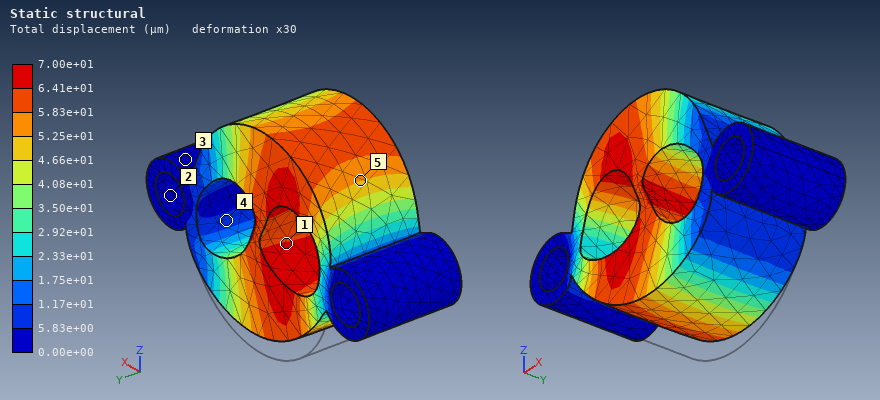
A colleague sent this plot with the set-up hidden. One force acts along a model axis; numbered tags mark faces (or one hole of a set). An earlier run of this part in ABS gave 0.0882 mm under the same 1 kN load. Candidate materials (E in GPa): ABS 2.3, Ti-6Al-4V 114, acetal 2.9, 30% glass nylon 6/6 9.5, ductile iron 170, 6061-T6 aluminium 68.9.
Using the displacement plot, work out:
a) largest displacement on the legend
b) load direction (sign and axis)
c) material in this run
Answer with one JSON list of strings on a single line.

["7.00e+01 µm", "+Z", "acetal"]
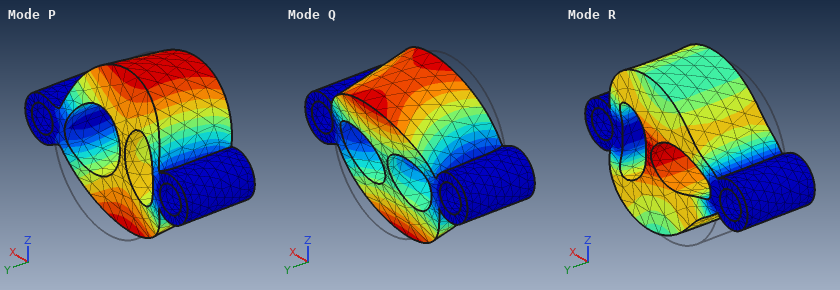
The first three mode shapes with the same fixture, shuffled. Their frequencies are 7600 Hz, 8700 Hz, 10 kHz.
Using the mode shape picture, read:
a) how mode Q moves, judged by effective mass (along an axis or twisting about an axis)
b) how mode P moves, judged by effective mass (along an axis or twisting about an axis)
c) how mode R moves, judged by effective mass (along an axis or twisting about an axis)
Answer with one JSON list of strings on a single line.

["twisting about X", "along Y", "along X"]
